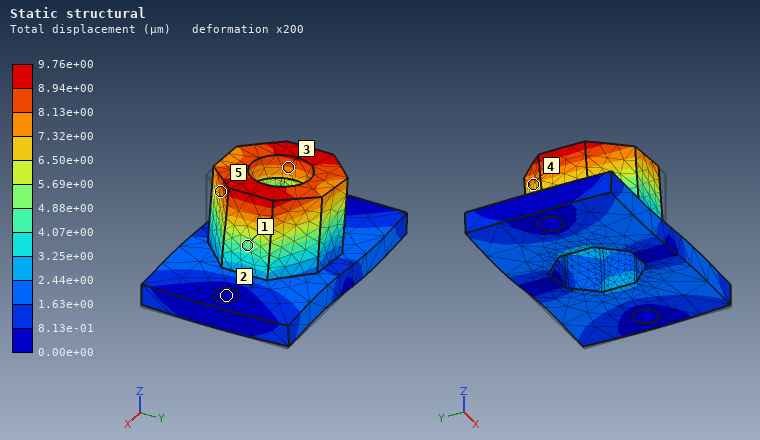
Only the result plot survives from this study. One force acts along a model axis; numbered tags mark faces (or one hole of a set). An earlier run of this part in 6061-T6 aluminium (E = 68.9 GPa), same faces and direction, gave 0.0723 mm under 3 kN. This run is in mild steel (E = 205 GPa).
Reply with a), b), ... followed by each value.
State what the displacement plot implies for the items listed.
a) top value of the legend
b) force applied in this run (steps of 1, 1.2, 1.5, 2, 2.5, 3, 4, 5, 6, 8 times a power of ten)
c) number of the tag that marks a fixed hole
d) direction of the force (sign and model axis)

a) 9.76e+00 µm
b) 1.2 kN
c) 2
d) -X
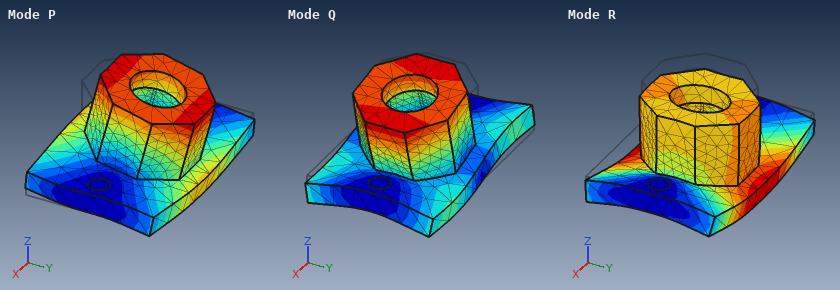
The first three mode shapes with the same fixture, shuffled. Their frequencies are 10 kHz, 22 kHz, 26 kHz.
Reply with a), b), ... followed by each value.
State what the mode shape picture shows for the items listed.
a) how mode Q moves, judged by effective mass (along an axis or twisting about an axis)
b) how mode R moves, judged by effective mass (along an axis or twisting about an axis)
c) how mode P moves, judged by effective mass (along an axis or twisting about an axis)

a) along X
b) along Z
c) along Y
